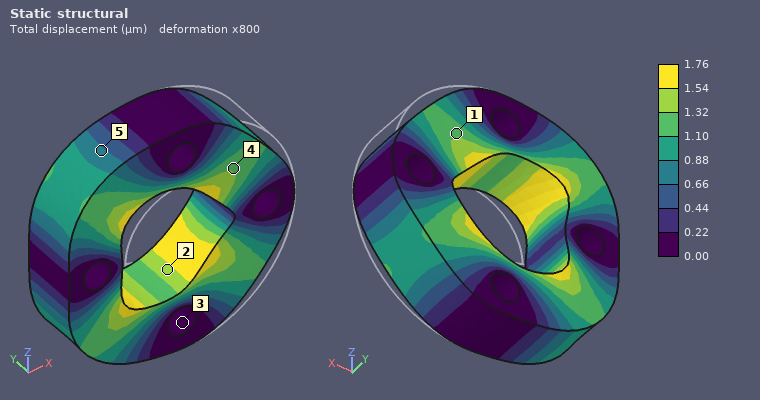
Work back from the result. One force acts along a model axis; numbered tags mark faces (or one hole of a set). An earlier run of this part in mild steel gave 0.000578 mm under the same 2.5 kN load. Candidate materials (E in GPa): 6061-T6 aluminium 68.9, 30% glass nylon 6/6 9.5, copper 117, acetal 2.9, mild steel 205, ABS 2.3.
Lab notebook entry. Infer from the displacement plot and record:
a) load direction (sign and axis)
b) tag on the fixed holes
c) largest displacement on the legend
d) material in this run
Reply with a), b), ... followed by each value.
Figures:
a) -X
b) 3
c) 1.76 µm
d) 6061-T6 aluminium
